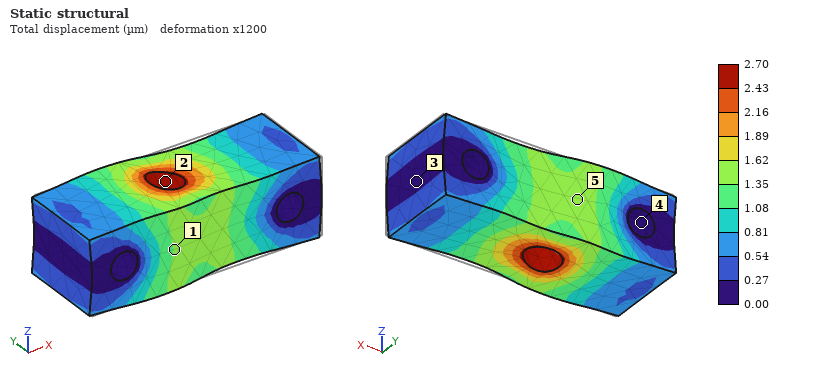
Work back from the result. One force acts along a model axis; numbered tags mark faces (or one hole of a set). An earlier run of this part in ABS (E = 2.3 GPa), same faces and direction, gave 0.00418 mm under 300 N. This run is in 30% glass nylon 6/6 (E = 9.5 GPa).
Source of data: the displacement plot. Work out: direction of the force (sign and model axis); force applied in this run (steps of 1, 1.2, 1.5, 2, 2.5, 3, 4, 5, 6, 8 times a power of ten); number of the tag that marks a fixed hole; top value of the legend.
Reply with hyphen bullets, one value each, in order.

- -X
- 800 N
- 4
- 2.70 µm
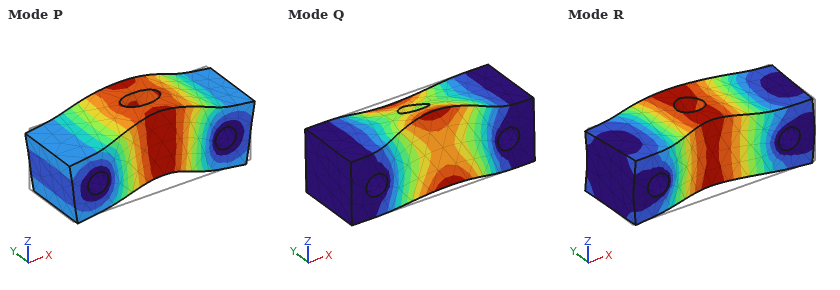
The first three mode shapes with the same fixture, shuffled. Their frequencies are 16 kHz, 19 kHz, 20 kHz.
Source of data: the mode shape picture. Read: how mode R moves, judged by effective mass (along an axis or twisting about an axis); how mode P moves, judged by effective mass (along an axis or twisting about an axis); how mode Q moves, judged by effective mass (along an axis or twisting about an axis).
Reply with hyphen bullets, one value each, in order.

- along Y
- along Z
- twisting about X
